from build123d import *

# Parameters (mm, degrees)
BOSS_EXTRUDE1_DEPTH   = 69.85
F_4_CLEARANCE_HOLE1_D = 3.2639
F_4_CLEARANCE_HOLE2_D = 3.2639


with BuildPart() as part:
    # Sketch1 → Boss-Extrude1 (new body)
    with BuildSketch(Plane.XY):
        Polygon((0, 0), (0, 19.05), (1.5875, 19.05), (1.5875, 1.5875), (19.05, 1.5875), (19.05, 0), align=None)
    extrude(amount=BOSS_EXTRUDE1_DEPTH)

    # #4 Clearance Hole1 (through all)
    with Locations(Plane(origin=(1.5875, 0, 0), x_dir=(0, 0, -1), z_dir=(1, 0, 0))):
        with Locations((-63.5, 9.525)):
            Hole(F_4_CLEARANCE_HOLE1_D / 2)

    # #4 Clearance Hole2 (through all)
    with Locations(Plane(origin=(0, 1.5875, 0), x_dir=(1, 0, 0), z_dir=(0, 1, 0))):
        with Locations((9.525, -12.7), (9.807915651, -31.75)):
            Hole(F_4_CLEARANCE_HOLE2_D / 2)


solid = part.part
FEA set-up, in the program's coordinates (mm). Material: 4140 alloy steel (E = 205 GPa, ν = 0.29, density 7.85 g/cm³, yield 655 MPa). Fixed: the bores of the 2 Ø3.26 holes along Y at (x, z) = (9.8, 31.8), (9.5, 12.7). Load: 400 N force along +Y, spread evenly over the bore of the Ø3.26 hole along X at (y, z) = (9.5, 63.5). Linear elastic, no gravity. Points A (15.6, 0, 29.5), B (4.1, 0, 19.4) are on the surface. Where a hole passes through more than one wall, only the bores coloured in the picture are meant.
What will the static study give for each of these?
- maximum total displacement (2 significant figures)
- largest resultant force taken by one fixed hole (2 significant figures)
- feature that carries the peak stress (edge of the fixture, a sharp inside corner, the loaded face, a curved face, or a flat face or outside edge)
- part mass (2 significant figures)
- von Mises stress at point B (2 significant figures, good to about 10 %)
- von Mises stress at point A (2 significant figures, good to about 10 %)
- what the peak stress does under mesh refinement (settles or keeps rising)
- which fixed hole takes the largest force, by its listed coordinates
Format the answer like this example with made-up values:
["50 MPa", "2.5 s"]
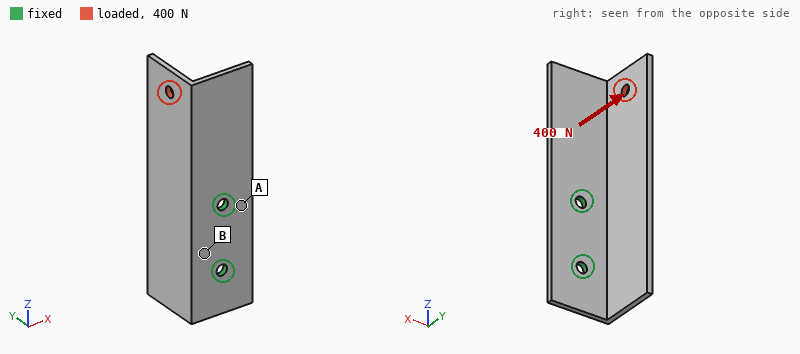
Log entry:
["0.52 mm", "910 N", "edge of the fixture", "31 g", "190 MPa", "89 MPa", "keeps rising", "(9.8, 31.8)"]
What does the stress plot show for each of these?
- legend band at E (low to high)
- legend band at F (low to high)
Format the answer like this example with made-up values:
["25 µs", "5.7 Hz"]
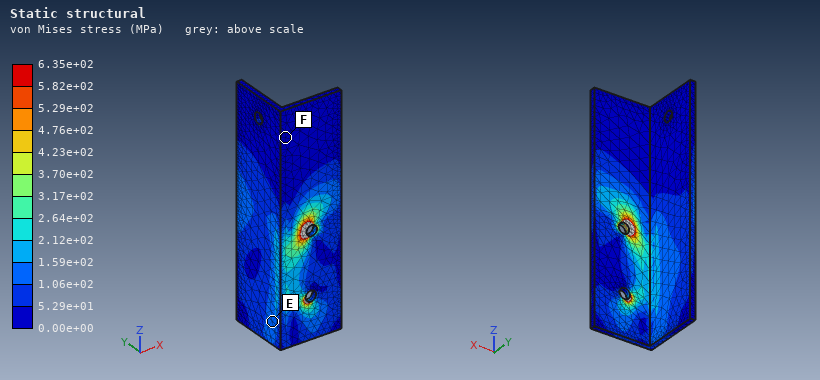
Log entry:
["1.06e+02 to 1.59e+02 MPa", "0.00e+00 to 5.29e+01 MPa"]
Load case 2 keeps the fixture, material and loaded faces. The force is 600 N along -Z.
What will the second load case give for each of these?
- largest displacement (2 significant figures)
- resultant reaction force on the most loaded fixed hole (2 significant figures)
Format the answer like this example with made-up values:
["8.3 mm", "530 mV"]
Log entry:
["0.13 mm", "460 N"]
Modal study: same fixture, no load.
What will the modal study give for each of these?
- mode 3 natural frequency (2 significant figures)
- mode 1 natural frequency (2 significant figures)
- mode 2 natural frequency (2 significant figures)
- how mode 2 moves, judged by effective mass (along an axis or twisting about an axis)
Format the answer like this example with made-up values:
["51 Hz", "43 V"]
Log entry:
["2700 Hz", "1600 Hz", "1900 Hz", "along Y"]
